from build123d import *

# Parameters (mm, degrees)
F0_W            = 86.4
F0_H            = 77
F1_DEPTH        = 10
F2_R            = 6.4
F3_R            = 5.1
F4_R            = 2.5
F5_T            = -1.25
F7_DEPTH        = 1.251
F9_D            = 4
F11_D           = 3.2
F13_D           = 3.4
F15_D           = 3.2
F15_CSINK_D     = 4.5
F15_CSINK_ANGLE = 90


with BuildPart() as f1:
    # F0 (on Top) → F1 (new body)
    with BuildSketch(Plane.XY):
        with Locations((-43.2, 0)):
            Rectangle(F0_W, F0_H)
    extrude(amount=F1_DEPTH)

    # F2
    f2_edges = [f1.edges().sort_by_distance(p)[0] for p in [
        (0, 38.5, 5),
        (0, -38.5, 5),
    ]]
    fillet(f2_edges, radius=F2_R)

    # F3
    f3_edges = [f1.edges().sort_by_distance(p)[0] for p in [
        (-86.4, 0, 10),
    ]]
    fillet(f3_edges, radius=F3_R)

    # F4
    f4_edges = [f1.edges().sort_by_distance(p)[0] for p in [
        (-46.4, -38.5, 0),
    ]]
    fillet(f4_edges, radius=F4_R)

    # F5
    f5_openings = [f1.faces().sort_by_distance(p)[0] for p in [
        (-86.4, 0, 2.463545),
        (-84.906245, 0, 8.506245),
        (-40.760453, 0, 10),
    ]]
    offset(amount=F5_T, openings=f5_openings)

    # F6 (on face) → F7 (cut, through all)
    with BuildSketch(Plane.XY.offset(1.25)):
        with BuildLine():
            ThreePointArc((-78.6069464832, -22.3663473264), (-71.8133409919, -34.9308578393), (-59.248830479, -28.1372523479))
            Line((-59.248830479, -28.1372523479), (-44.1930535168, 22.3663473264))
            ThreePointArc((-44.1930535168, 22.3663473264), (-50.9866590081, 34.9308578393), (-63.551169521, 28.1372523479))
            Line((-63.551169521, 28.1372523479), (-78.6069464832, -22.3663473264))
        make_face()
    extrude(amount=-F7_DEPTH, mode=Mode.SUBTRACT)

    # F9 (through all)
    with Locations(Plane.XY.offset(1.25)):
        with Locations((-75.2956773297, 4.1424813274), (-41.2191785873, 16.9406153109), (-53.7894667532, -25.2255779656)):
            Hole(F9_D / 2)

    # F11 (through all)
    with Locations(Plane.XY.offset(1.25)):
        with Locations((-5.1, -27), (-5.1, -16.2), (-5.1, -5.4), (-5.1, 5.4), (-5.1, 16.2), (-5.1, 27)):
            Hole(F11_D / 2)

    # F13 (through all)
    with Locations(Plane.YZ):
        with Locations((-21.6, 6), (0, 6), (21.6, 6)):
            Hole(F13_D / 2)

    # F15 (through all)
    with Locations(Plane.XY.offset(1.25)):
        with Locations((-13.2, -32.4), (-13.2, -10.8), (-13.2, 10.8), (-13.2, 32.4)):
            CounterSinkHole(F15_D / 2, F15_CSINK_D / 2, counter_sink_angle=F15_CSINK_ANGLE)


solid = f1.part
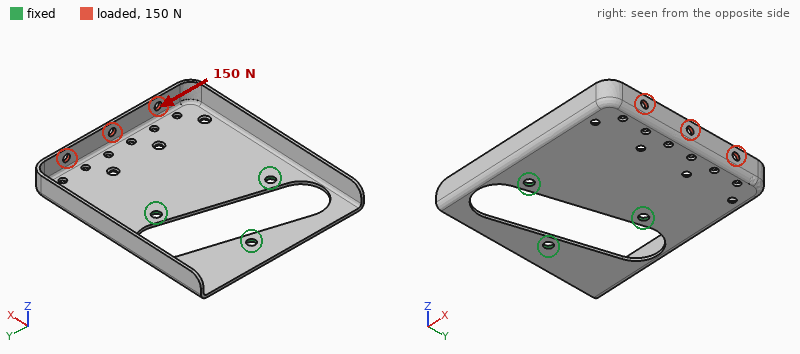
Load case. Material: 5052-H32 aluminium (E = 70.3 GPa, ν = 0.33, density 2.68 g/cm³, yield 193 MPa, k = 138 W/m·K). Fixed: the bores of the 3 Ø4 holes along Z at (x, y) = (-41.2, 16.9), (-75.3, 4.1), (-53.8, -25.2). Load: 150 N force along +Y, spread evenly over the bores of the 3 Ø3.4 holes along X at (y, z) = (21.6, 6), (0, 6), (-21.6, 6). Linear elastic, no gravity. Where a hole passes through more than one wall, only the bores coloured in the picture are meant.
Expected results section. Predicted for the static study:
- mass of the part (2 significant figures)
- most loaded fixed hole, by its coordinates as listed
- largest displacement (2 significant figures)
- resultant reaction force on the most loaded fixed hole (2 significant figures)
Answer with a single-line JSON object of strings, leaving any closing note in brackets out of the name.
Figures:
{"mass of the part": "23 g", "most loaded fixed hole, by its coordinates as listed": "(-41.2, 16.9)", "largest displacement": "0.45 mm", "resultant reaction force on the most loaded fixed hole": "180 N"}
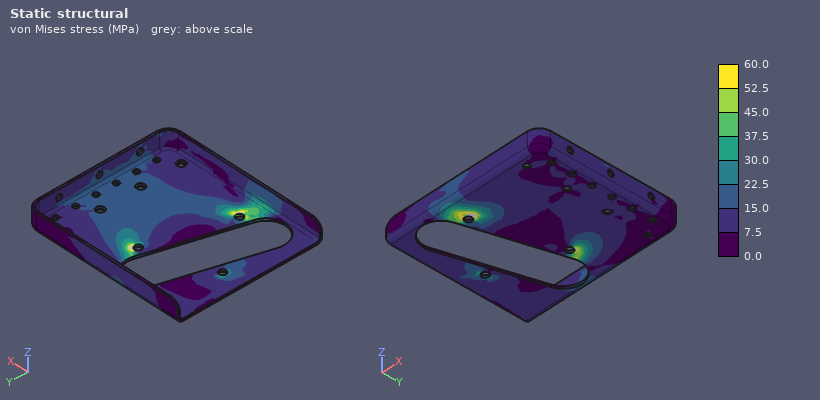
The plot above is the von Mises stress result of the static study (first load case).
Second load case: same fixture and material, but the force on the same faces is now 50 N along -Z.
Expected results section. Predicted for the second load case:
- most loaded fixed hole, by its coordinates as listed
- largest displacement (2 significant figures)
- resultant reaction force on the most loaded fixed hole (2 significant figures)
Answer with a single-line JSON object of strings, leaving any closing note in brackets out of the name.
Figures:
{"most loaded fixed hole, by its coordinates as listed": "(-41.2, 16.9)", "largest displacement": "0.92 mm", "resultant reaction force on the most loaded fixed hole": "47 N"}
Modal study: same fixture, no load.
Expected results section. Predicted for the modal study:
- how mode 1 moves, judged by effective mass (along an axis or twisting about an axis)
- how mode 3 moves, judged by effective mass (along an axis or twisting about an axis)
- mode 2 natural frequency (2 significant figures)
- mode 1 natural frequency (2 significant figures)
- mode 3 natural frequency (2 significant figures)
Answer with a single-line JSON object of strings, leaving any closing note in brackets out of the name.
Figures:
{"how mode 1 moves, judged by effective mass": "along Z", "how mode 3 moves, judged by effective mass": "along Z", "mode 2 natural frequency": "690 Hz", "mode 1 natural frequency": "480 Hz", "mode 3 natural frequency": "850 Hz"}
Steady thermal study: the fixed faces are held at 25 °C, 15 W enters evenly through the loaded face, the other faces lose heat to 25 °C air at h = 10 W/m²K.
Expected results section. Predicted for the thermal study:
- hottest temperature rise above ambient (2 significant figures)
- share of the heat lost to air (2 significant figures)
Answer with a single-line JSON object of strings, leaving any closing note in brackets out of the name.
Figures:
{"hottest temperature rise above ambient": "64 K", "share of the heat lost to air": "21 %"}
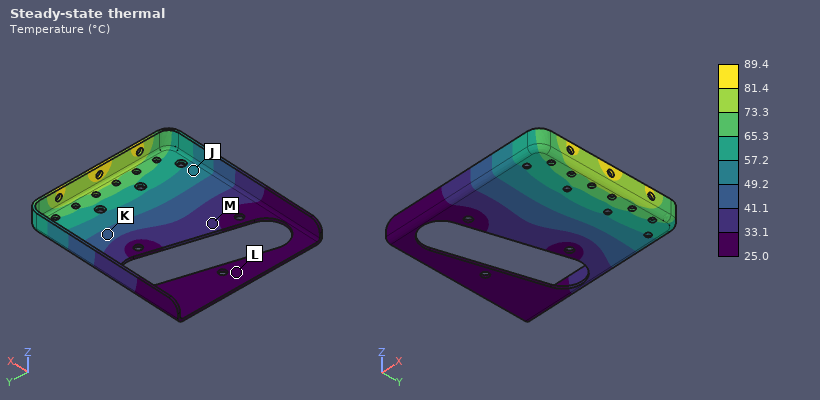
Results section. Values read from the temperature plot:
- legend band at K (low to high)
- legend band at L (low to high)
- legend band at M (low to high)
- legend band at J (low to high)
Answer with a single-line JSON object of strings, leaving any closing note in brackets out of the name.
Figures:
{"legend band at K": "41.1 to 49.2 °C", "legend band at L": "25.0 to 33.1 °C", "legend band at M": "33.1 to 41.1 °C", "legend band at J": "49.2 to 57.2 °C"}
